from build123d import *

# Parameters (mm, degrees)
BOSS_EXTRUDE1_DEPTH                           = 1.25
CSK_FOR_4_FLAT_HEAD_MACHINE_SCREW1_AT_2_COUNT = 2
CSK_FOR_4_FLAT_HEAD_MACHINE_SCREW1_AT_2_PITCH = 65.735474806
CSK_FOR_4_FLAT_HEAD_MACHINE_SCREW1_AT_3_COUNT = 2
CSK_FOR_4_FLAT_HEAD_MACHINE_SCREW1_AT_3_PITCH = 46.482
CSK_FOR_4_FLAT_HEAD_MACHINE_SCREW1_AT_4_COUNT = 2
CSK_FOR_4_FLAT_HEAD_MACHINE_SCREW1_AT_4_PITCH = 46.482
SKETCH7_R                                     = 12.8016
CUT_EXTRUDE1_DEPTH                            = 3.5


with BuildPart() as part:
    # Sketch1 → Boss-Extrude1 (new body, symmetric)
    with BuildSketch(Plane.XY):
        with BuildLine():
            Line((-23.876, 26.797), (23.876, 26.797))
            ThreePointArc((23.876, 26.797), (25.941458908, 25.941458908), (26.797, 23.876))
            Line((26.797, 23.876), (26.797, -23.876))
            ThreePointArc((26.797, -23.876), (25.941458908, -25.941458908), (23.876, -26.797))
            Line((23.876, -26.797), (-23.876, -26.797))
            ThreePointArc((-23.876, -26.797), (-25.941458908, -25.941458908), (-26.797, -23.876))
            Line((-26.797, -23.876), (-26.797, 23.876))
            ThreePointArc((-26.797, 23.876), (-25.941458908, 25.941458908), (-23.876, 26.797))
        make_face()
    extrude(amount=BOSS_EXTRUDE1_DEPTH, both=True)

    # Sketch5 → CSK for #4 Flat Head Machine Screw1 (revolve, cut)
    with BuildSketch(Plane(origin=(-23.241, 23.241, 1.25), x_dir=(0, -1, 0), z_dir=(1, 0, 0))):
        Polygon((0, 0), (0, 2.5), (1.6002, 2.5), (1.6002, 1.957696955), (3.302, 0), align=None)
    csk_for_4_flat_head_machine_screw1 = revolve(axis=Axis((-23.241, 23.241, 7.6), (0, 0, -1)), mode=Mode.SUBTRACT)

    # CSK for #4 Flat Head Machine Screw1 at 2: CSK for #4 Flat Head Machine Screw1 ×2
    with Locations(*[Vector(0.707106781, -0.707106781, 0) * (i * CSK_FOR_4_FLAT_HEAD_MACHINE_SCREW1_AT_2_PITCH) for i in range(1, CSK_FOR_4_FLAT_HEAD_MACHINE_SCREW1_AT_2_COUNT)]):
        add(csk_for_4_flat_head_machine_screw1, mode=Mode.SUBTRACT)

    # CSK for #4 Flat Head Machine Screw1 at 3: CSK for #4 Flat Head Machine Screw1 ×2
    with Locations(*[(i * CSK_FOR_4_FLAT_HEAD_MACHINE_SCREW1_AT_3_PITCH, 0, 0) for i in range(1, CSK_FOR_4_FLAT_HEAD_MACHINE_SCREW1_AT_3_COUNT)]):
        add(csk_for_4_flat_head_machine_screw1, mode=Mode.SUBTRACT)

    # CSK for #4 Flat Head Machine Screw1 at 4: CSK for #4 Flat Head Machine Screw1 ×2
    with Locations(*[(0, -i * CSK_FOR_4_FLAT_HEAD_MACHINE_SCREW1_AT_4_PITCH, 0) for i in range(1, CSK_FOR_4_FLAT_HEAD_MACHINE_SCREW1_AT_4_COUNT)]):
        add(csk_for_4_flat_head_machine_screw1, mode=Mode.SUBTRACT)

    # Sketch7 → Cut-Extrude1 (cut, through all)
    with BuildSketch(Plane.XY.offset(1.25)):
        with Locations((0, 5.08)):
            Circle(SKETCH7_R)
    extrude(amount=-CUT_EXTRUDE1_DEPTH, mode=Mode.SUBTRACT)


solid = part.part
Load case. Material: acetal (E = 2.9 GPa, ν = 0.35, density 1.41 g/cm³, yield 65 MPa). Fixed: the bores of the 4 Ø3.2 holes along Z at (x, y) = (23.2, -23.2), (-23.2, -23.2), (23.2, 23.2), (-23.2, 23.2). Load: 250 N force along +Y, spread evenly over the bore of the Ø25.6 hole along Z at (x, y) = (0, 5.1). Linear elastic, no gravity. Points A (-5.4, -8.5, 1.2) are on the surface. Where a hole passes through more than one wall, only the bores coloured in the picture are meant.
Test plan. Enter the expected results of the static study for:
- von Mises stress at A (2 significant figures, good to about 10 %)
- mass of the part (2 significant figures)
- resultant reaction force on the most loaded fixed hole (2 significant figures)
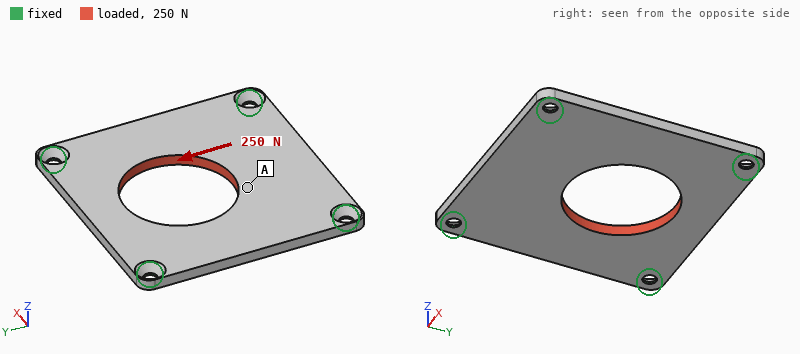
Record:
1.4 MPa
8.0 g
65 N
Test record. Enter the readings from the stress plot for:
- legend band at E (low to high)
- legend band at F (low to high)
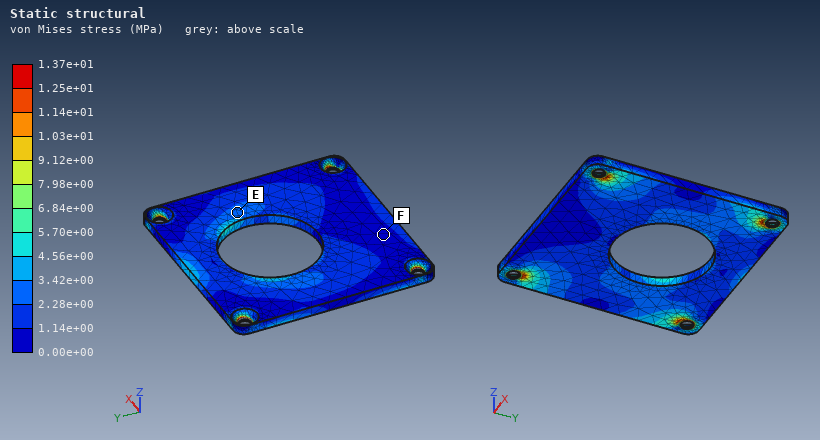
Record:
2.28e+00 to 3.42e+00 MPa
0.00e+00 to 1.14e+00 MPa
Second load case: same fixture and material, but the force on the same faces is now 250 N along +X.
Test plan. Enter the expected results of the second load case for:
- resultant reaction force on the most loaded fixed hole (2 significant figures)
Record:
68 N
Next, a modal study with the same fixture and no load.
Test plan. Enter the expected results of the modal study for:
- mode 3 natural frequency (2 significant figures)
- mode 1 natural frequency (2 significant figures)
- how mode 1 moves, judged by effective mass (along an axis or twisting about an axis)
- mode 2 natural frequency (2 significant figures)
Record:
1500 Hz
990 Hz
along Z
1500 Hz
